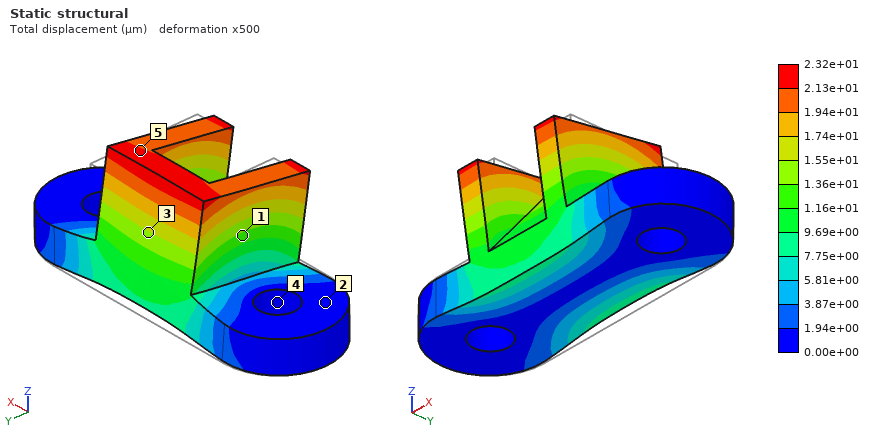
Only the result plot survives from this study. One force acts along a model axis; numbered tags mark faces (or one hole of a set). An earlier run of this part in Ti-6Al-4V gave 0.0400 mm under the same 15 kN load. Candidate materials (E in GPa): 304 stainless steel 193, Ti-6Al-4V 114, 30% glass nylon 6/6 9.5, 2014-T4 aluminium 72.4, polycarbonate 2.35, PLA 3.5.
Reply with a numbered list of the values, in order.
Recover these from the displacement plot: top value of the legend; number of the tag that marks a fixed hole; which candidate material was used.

1. 2.32e+01 µm
2. 4
3. 304 stainless steel
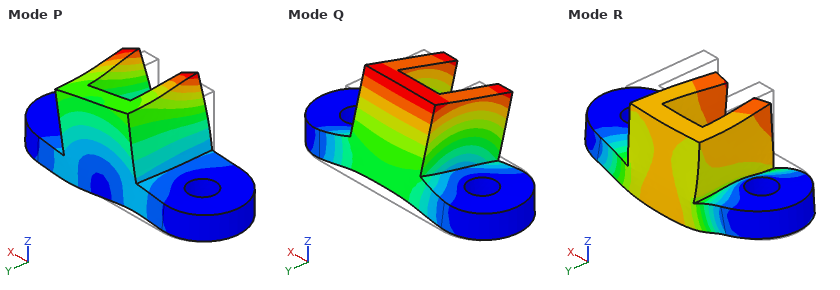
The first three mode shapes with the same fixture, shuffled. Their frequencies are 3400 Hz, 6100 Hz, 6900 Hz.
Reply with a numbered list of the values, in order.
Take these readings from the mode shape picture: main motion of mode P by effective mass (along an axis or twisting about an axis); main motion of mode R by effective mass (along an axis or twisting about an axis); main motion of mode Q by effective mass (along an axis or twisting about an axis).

1. along X
2. along Z
3. along Y
